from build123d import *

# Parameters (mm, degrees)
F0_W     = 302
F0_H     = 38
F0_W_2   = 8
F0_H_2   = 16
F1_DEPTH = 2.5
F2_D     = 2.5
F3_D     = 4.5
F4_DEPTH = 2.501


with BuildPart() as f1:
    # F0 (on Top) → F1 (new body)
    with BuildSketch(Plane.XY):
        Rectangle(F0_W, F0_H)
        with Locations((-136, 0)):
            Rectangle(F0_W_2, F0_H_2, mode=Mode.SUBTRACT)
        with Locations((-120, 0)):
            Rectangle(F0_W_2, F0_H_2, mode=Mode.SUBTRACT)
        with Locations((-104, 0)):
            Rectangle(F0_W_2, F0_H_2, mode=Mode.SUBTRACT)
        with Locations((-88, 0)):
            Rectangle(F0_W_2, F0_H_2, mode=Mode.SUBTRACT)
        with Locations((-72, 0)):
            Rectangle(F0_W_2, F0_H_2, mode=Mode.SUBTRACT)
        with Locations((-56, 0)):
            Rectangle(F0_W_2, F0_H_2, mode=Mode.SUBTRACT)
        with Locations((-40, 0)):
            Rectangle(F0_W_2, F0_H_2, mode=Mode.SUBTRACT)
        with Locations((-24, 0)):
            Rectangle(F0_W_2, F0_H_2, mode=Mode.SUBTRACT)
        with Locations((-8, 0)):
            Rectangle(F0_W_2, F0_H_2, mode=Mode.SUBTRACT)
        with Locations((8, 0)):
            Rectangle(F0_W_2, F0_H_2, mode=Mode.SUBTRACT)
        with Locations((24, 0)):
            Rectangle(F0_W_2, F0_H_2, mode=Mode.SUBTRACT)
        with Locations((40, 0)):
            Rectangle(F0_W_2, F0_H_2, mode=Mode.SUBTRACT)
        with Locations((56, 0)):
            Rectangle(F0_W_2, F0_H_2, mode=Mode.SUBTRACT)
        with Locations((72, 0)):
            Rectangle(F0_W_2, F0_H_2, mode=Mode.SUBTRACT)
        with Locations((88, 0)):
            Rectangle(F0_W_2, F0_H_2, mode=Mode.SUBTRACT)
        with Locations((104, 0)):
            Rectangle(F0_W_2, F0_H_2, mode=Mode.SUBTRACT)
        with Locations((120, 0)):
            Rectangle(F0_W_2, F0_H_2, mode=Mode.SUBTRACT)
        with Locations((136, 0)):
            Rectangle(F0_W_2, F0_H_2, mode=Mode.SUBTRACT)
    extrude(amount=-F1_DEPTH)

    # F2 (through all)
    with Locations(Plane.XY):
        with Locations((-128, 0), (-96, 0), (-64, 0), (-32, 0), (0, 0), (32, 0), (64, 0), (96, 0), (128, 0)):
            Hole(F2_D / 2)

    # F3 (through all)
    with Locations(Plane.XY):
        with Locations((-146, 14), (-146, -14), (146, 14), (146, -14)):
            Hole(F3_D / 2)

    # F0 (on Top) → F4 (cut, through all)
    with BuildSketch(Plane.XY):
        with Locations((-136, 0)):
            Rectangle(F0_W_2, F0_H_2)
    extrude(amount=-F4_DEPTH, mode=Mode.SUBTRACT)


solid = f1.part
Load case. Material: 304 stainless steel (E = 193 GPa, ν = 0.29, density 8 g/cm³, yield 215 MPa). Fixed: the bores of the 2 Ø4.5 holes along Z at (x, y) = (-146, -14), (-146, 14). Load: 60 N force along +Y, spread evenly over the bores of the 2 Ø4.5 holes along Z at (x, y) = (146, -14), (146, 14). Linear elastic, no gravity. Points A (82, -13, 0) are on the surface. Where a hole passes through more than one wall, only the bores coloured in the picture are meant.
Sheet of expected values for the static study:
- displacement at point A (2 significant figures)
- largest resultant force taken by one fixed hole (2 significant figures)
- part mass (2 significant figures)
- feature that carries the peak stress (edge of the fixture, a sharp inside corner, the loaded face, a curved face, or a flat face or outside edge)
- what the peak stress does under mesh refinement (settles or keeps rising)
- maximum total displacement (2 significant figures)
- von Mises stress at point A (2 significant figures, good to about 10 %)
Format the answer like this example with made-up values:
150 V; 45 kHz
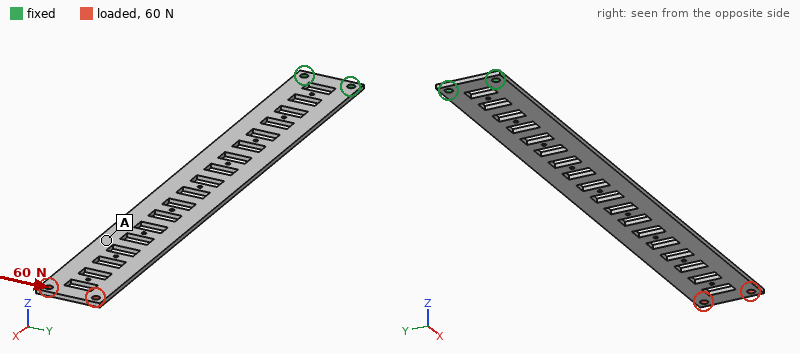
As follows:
0.18 mm; 590 N; 180 g; edge of the fixture; keeps rising; 0.27 mm; 6.0 MPa
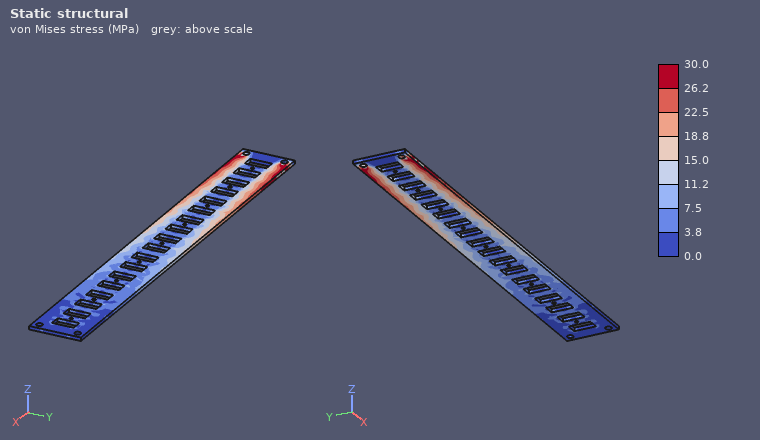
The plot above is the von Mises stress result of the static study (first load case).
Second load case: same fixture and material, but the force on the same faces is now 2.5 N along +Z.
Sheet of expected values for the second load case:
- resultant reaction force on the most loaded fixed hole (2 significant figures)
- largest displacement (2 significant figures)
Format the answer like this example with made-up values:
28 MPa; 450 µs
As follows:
1.3 N; 3.6 mm
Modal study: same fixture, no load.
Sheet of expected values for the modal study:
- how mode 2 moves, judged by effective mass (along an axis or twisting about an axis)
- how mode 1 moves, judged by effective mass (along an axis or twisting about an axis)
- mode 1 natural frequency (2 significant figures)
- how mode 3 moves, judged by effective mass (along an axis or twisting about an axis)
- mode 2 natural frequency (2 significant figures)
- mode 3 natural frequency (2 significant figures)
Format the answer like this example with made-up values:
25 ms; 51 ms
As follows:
along Z; along Z; 20 Hz; twisting about X; 130 Hz; 300 Hz
